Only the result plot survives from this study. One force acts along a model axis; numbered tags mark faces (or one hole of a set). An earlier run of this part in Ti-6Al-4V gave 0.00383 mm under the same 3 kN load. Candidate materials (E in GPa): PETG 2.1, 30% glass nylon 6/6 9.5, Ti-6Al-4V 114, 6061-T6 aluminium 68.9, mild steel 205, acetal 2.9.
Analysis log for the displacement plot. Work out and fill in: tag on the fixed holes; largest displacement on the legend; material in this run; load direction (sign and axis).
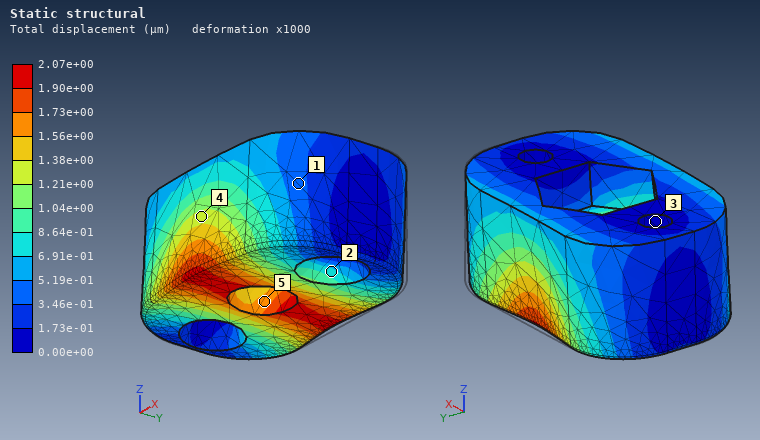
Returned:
3
2.07e+00 µm
mild steel
-Y
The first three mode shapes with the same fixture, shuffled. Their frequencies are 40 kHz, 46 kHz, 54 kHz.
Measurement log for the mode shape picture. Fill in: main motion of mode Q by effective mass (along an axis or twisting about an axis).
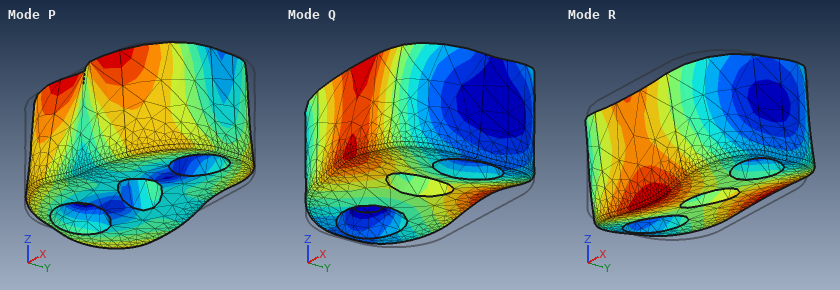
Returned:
along Z
